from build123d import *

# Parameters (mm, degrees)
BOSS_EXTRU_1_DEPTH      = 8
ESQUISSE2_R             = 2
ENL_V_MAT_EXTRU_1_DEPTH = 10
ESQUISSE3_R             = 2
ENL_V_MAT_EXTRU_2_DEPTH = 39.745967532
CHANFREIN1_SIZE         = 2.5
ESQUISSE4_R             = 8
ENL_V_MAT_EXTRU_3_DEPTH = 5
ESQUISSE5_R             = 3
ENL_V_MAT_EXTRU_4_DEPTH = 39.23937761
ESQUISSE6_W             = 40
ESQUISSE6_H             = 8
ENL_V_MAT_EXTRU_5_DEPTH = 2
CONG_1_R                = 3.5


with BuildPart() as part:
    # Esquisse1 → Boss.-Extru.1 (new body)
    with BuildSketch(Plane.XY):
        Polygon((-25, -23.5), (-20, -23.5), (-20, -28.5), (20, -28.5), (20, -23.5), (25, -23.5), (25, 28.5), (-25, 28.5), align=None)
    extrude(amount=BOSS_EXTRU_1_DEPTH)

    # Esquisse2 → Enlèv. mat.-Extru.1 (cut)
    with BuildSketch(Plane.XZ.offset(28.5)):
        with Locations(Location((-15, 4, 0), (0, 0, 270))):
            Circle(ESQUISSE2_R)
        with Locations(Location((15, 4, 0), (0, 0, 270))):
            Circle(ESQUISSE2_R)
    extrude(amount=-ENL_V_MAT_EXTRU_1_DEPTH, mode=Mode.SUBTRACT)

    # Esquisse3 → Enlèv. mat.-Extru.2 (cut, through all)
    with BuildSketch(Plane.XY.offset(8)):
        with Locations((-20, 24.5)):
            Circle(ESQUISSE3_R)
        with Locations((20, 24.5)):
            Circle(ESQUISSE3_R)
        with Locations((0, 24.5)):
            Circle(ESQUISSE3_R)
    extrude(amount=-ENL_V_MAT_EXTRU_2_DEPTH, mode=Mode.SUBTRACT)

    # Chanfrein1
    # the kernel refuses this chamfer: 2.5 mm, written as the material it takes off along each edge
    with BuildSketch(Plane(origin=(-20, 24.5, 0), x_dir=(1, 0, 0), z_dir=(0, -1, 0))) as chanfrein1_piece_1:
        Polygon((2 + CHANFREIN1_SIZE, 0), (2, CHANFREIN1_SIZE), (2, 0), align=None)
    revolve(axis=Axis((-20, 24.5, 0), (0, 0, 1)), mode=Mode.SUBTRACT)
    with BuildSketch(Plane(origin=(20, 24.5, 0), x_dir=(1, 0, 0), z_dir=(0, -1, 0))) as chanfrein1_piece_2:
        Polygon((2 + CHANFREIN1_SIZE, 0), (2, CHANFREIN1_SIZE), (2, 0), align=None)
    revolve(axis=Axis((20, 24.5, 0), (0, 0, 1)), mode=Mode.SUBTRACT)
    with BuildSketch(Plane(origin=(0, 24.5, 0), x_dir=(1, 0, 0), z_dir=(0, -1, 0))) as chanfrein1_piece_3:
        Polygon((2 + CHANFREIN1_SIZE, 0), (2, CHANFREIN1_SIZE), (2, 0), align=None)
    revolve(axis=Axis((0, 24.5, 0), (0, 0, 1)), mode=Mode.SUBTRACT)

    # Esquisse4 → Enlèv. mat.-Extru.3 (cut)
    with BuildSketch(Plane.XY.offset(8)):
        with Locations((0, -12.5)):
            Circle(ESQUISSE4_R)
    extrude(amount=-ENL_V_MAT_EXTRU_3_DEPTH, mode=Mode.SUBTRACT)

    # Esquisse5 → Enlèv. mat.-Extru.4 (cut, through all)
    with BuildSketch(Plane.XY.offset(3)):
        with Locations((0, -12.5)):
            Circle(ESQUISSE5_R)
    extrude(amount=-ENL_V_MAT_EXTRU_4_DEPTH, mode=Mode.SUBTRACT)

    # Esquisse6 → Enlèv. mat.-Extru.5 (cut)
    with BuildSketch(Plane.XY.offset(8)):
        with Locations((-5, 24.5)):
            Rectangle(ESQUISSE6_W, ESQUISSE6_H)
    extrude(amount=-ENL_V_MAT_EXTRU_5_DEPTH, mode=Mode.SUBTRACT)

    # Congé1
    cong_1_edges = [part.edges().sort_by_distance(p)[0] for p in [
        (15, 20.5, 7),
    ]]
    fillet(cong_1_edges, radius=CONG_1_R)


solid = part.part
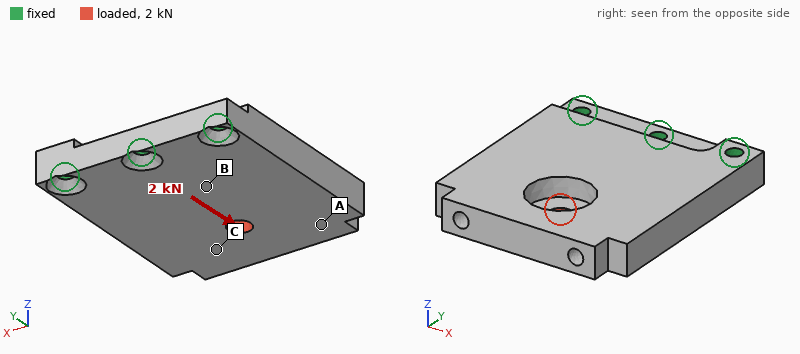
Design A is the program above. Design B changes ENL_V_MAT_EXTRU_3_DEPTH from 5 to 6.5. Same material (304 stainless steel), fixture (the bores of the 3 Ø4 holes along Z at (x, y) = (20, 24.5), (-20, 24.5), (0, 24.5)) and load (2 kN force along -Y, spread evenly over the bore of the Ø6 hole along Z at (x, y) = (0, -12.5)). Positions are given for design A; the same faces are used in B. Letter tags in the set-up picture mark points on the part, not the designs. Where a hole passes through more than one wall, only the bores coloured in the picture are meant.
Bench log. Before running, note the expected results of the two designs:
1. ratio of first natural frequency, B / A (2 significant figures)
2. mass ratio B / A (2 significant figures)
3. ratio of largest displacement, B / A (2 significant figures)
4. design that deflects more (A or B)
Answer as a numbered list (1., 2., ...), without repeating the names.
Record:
1. 1.0
2. 0.99
3. 1.3
4. B
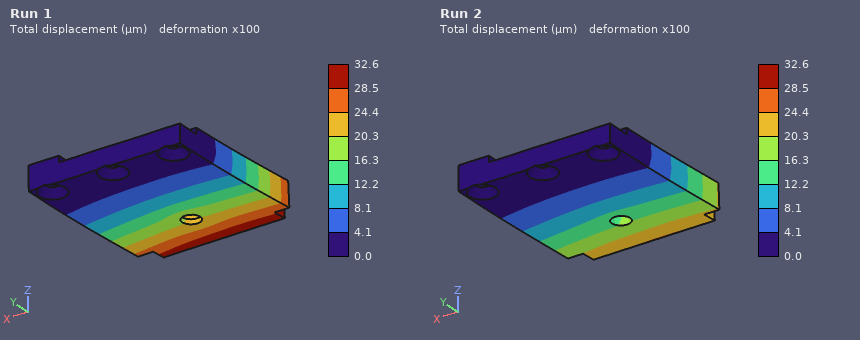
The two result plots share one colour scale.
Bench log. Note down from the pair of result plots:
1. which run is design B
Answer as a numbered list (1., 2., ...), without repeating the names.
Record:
1. Run 1
